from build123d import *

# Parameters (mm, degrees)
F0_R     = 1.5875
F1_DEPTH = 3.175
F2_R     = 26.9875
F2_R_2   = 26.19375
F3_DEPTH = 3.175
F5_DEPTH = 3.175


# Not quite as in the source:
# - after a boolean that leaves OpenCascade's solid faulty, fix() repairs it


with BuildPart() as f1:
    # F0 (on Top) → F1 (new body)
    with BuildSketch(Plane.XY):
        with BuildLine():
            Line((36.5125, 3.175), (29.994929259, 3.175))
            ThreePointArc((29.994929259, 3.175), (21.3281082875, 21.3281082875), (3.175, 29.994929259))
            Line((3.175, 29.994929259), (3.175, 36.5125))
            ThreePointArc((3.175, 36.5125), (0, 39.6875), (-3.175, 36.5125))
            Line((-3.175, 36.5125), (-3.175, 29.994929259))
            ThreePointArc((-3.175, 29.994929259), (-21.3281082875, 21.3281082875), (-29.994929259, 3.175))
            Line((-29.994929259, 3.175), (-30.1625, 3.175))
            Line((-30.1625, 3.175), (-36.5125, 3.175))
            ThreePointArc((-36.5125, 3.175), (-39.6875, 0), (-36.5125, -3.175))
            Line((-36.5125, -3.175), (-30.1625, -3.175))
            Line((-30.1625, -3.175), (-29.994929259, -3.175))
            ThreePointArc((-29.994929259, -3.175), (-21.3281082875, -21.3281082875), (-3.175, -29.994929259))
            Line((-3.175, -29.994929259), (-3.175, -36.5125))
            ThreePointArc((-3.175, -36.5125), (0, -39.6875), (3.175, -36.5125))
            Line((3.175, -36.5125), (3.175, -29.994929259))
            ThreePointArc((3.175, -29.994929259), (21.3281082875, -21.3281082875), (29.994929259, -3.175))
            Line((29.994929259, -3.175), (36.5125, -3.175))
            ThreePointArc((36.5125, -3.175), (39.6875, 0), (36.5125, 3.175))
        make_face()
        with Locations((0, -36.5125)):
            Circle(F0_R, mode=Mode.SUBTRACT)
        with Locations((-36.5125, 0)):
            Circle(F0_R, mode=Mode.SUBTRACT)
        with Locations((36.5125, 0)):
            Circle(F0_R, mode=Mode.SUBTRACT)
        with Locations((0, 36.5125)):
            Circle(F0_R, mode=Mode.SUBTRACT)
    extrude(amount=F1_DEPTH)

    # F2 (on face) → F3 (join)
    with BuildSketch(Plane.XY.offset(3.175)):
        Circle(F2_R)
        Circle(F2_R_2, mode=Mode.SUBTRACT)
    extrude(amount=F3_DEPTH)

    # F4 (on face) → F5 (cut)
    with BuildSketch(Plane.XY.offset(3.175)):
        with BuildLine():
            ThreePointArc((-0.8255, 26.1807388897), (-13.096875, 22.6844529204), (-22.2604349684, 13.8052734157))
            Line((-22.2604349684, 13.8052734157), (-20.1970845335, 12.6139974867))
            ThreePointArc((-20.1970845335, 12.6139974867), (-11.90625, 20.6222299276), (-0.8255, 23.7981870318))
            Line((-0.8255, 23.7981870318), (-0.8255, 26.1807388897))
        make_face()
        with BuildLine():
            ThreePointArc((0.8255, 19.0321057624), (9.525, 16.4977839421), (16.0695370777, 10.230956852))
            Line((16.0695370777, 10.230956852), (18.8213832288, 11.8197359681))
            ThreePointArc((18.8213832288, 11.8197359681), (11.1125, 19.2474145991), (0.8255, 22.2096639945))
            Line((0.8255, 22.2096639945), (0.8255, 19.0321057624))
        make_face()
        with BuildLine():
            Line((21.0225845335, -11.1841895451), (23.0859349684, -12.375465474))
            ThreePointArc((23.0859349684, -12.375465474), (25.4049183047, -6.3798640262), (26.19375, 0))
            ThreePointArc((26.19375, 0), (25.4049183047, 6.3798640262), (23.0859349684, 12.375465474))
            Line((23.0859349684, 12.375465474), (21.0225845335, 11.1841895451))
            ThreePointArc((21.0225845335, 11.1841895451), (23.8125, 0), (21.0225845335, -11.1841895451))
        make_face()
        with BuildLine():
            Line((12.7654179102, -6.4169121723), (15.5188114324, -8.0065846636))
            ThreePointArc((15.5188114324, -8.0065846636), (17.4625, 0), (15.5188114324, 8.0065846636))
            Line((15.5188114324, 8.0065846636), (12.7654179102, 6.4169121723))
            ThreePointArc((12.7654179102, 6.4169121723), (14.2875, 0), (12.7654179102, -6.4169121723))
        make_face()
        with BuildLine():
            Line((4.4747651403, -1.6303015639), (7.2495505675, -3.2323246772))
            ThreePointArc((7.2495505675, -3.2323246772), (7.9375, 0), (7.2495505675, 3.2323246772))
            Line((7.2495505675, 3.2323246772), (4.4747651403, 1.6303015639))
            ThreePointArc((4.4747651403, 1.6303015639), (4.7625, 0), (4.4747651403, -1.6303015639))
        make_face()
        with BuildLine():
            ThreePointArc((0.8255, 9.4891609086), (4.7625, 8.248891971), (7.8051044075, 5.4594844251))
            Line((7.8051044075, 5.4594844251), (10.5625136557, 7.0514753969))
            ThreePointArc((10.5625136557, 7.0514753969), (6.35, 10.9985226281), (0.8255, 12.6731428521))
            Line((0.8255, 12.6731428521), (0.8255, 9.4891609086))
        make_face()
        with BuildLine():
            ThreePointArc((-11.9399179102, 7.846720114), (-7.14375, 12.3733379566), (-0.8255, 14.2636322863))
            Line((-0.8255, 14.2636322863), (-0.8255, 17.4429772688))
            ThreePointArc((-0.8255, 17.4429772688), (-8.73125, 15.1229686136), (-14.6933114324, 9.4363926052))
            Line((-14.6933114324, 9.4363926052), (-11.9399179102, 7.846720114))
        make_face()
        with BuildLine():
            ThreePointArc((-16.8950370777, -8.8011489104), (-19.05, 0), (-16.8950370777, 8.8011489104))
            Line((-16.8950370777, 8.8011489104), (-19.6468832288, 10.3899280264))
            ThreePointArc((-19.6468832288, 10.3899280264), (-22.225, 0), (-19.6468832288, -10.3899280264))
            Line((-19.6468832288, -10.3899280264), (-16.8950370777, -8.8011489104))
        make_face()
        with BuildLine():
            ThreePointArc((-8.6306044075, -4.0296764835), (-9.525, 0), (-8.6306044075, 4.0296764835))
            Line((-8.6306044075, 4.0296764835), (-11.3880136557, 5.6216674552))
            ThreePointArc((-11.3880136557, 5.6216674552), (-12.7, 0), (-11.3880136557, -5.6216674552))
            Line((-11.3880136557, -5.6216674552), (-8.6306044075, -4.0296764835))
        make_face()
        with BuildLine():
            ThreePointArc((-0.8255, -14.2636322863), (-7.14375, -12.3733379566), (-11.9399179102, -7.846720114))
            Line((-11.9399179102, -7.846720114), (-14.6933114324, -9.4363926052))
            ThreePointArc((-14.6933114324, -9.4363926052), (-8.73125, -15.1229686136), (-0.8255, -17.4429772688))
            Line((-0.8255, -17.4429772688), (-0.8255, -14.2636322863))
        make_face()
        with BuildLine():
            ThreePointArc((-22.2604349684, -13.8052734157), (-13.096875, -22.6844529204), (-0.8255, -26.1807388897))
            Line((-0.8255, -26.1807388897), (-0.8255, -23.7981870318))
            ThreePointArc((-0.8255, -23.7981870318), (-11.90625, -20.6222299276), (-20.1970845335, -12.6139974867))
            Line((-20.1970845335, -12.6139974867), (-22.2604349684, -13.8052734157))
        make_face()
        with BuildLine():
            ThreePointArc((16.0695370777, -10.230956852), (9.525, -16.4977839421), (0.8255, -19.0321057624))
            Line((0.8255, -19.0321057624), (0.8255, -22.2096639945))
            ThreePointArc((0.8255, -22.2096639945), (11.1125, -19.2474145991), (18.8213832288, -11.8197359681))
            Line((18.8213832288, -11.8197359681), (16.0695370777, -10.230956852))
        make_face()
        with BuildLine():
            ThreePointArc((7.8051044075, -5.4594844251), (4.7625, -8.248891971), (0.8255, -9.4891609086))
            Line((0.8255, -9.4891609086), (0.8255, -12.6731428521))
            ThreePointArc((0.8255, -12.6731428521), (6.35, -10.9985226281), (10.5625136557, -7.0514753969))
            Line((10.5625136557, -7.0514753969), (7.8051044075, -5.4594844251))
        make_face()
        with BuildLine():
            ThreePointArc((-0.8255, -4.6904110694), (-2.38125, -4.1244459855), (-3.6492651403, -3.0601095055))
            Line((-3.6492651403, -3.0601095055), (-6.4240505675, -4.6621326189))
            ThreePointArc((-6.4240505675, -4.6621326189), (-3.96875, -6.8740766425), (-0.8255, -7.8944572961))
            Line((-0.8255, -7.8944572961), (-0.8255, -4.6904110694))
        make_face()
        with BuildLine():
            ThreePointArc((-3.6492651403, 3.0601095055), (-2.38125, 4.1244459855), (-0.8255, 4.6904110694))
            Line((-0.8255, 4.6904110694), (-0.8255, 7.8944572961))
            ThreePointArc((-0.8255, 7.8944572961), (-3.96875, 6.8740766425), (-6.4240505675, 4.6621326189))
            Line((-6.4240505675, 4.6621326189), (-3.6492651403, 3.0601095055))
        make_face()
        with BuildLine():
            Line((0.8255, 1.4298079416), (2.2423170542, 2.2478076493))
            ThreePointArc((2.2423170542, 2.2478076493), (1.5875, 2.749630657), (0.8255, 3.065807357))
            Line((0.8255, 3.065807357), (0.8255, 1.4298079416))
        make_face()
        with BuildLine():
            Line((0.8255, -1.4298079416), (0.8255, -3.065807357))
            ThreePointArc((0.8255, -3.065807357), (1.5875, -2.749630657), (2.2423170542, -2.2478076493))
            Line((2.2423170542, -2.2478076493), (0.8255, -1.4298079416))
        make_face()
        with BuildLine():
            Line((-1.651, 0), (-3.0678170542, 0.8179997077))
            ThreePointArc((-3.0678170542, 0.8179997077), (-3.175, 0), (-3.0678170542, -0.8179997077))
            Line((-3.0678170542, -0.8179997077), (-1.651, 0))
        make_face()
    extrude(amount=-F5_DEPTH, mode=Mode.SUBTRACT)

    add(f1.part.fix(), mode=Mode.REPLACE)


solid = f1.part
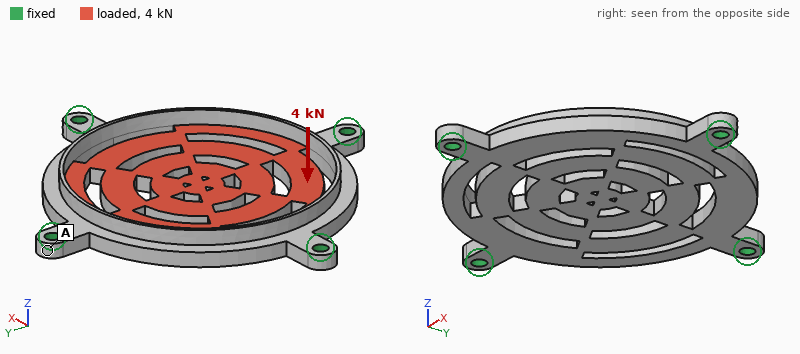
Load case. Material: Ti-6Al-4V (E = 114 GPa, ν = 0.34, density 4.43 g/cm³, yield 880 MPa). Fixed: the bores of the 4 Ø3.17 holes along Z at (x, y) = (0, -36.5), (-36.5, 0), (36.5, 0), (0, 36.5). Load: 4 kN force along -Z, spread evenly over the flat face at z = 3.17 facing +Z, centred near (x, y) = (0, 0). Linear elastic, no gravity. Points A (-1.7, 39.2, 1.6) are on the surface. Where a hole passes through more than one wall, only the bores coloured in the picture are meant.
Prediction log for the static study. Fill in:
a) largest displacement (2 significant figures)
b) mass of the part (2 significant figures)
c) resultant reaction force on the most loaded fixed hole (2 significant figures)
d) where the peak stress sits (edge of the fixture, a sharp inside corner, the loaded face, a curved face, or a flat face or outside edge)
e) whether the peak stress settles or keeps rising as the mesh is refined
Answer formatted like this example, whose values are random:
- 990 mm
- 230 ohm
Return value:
- 0.47 mm
- 36 g
- 1.1 kN
- edge of the fixture
- keeps rising
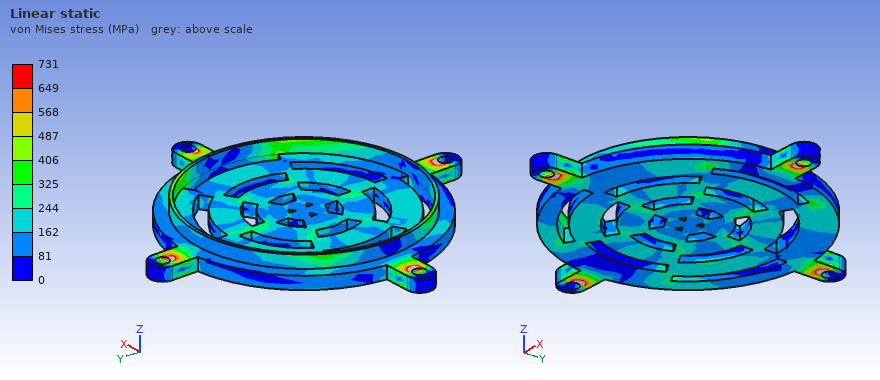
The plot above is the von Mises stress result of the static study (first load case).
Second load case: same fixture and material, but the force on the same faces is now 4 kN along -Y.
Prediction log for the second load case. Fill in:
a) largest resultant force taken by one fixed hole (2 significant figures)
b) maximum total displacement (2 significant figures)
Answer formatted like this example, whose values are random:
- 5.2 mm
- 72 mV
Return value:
- 1.4 kN
- 31 µm
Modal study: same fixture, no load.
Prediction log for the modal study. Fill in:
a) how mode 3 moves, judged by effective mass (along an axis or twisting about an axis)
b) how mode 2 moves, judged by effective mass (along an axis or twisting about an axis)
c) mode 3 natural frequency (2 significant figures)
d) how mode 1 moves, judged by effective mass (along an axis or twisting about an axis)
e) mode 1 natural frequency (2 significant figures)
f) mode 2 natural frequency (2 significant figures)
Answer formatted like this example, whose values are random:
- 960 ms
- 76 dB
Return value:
- twisting about X
- twisting about Y
- 5600 Hz
- along Z
- 3500 Hz
- 5400 Hz
